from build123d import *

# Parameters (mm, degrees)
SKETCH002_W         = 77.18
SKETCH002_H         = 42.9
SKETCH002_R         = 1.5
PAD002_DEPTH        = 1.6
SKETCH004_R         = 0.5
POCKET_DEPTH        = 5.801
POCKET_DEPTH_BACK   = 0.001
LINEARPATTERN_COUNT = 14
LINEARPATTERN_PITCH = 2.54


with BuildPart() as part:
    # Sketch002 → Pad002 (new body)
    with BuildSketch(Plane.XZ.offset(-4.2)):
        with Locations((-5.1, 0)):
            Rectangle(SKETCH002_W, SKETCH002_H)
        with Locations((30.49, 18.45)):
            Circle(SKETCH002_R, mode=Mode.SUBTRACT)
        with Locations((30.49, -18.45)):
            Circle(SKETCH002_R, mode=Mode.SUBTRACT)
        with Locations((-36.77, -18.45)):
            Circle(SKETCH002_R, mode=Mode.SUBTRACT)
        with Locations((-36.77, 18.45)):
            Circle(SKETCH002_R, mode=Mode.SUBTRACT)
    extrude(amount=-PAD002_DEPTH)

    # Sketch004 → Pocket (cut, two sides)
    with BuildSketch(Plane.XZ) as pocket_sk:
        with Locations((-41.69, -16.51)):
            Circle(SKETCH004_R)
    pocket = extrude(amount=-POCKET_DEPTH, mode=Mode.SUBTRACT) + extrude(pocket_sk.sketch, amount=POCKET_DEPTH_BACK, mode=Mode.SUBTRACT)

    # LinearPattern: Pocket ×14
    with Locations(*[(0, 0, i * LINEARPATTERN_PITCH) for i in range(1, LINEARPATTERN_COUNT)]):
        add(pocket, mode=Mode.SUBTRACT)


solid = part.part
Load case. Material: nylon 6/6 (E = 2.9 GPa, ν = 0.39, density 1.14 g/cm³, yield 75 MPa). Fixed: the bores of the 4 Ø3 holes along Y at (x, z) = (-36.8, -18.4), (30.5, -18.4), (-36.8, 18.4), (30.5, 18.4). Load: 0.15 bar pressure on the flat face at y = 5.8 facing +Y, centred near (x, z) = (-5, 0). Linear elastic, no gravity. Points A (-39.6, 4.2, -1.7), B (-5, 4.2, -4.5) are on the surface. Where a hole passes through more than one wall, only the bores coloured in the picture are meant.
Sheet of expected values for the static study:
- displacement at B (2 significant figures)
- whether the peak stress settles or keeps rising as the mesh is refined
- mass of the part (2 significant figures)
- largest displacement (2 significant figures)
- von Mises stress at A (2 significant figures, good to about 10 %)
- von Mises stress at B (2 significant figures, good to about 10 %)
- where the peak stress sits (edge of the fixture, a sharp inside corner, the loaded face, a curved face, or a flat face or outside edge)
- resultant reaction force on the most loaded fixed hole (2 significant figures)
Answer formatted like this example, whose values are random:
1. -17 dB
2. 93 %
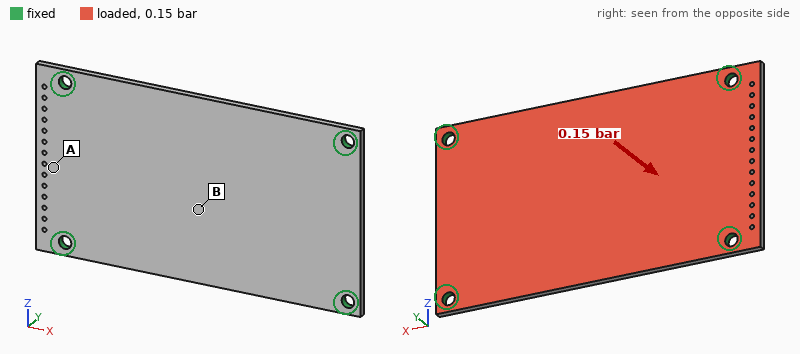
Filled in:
1. 0.98 mm
2. keeps rising
3. 6.0 g
4. 1.0 mm
5. 2.2 MPa
6. 6.5 MPa
7. edge of the fixture
8. 13 N
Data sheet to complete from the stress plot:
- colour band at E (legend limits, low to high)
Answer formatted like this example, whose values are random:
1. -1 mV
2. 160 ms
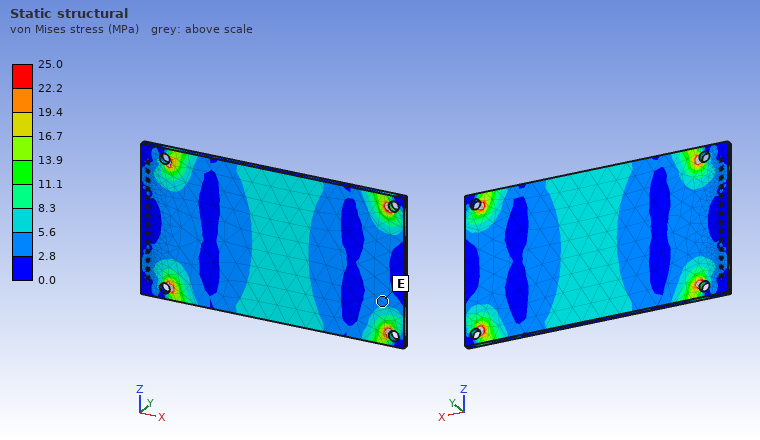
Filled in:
1. 2.8 to 5.6 MPa
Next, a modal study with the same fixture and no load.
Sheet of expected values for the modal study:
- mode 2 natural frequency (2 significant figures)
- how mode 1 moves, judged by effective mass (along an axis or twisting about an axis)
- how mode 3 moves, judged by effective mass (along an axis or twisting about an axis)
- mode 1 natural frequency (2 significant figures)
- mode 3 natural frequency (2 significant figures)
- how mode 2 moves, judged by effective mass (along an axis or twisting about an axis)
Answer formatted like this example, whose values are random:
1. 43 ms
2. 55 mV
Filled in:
1. 850 Hz
2. along Y
3. twisting about Z
4. 520 Hz
5. 1400 Hz
6. twisting about X
